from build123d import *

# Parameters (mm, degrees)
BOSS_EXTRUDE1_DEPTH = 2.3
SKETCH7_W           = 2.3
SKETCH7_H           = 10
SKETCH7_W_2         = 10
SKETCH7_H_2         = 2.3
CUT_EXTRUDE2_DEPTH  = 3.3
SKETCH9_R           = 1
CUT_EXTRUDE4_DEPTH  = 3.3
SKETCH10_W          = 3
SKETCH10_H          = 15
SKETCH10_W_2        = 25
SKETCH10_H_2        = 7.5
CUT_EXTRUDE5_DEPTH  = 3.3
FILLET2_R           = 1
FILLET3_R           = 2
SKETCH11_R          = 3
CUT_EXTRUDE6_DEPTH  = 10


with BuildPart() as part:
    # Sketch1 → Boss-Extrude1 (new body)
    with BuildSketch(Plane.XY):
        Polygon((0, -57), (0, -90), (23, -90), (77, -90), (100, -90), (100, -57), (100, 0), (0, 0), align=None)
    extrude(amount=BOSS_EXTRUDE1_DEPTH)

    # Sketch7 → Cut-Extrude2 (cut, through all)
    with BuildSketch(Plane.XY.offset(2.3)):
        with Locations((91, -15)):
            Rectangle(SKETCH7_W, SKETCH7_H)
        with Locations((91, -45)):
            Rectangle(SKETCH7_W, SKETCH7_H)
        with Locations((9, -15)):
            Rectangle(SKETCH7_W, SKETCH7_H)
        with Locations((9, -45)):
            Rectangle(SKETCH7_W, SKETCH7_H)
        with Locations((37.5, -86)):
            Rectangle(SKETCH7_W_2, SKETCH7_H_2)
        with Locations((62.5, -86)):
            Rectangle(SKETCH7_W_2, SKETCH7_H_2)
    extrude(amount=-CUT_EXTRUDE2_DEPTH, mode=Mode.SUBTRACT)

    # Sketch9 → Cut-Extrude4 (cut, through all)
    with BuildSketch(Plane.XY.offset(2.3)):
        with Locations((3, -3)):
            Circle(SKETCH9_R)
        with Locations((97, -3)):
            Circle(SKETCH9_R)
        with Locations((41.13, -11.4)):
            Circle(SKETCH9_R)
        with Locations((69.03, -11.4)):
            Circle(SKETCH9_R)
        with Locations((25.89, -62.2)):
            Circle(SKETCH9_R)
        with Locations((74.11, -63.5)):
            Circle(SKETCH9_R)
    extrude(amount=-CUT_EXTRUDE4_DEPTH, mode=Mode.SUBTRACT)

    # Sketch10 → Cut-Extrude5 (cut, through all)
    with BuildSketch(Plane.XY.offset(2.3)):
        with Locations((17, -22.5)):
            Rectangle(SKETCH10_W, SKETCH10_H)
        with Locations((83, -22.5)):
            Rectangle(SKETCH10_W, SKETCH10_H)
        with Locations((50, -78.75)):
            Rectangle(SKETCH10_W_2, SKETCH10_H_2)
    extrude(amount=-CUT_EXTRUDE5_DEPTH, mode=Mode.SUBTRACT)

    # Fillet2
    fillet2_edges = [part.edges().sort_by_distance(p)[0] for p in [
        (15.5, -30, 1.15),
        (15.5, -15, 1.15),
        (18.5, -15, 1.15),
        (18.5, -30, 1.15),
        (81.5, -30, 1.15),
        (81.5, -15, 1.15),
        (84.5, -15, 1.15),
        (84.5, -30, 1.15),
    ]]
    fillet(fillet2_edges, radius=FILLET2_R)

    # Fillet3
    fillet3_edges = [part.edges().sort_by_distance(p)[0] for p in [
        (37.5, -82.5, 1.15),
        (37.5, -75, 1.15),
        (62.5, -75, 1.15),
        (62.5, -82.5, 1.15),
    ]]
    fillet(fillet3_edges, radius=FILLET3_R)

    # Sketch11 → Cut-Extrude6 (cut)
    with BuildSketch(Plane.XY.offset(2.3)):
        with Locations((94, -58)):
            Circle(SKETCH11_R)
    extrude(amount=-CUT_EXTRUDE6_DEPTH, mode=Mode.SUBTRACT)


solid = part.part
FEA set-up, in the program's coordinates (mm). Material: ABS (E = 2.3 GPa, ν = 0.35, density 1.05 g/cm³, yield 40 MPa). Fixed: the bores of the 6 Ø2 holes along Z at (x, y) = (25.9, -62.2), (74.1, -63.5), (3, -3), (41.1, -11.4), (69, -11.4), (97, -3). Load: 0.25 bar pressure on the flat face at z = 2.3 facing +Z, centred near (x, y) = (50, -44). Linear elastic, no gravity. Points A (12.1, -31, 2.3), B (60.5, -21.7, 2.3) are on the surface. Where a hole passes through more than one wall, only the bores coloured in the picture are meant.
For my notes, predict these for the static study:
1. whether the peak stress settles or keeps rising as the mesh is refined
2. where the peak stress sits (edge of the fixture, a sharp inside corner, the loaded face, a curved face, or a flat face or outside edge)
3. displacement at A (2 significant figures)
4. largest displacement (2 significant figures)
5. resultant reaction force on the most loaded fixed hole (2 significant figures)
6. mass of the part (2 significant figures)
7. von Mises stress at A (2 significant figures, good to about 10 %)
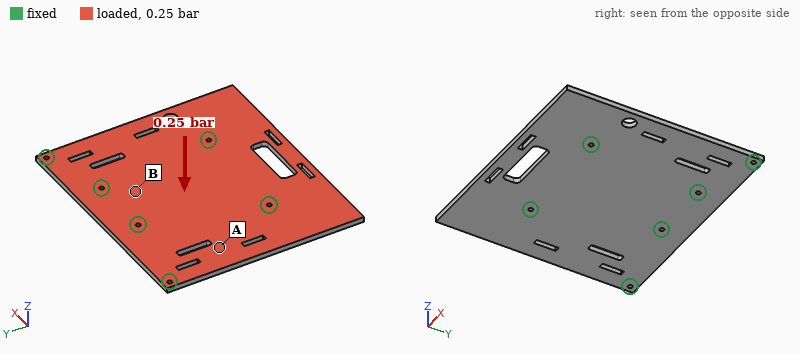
keeps rising
edge of the fixture
0.48 mm
1.5 mm
67 N
21 g
4.2 MPa
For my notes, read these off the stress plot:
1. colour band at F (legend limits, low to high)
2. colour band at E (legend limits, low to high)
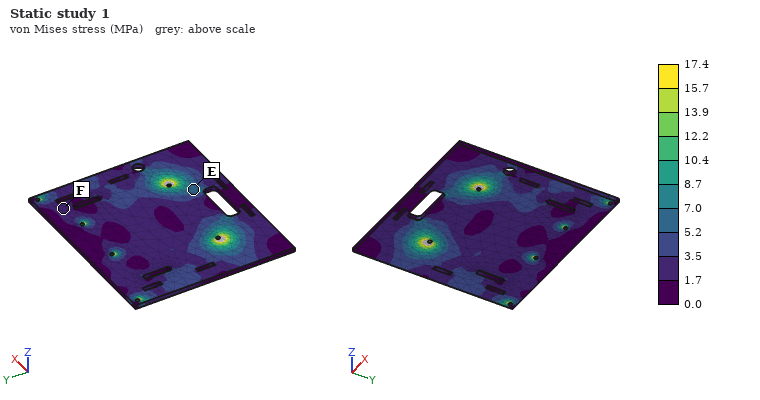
1.7 to 3.5 MPa
5.2 to 7.0 MPa
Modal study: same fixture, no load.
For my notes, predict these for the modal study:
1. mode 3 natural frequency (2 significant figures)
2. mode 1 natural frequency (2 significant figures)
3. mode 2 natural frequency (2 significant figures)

630 Hz
530 Hz
570 Hz
